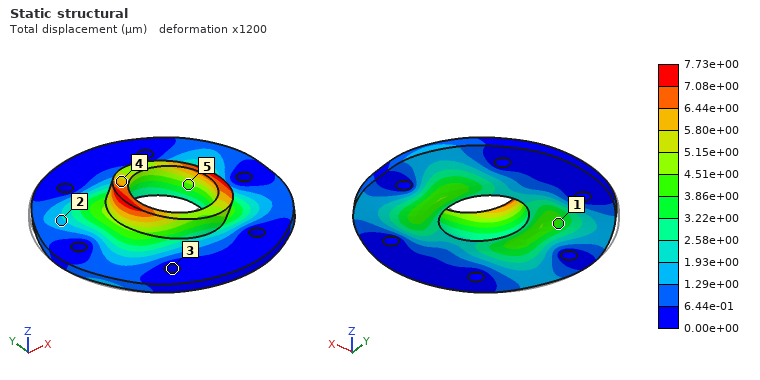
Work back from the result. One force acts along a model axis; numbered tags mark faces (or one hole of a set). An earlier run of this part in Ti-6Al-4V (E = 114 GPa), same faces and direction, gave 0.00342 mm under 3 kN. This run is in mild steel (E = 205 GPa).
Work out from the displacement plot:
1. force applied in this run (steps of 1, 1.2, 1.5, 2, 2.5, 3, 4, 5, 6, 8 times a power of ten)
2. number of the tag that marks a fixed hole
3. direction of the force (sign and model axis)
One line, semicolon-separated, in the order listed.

12 kN; 3; +X
